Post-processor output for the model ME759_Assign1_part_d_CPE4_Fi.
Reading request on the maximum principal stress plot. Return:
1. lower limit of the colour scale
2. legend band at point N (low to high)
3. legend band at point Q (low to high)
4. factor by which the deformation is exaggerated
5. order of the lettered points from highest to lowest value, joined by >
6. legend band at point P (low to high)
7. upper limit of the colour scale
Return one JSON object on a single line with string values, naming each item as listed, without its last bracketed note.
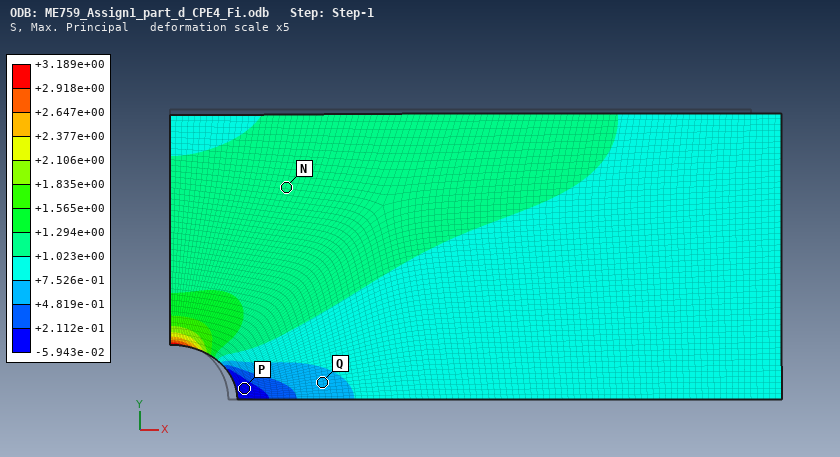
{"lower limit of the colour scale": "-5.943e-02", "legend band at point N": "+1.023e+00 to +1.294e+00", "legend band at point Q": "+4.819e-01 to +7.526e-01", "factor by which the deformation is exaggerated": "5", "order of the lettered points from highest to lowest value, joined by >": "N > Q > P", "legend band at point P": "-5.943e-02 to +2.112e-01", "upper limit of the colour scale": "+3.189e+00"}
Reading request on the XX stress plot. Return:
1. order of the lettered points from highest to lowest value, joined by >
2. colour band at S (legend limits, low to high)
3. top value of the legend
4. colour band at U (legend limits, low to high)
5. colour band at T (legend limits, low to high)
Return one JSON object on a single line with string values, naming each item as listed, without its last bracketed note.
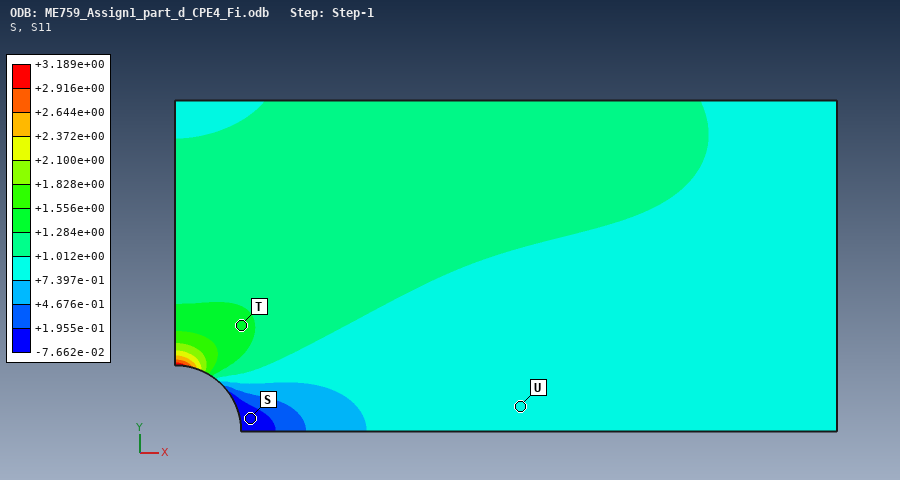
{"order of the lettered points from highest to lowest value, joined by >": "T > U > S", "colour band at S": "-7.662e-02 to +1.955e-01", "top value of the legend": "+3.189e+00", "colour band at U": "+7.397e-01 to +1.012e+00", "colour band at T": "+1.284e+00 to +1.556e+00"}
